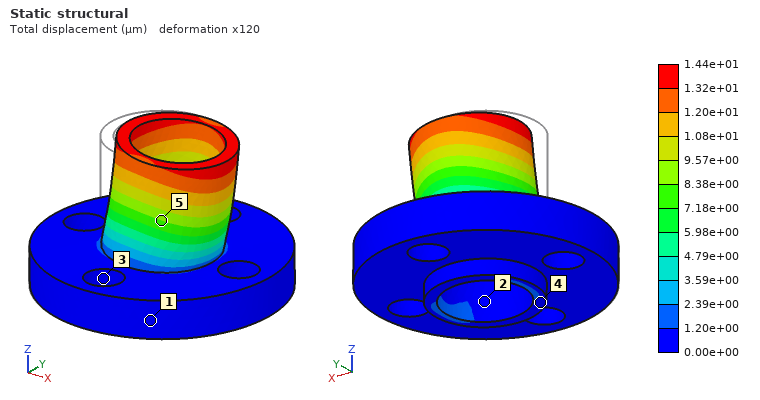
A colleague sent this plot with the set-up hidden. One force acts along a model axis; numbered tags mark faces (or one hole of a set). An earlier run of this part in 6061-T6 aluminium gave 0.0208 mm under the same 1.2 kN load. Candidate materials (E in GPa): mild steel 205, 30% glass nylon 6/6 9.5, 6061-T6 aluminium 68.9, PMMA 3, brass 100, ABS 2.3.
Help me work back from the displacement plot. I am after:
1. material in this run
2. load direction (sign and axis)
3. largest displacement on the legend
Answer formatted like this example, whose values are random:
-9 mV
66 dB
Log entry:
brass
+X
1.44e+01 µm
